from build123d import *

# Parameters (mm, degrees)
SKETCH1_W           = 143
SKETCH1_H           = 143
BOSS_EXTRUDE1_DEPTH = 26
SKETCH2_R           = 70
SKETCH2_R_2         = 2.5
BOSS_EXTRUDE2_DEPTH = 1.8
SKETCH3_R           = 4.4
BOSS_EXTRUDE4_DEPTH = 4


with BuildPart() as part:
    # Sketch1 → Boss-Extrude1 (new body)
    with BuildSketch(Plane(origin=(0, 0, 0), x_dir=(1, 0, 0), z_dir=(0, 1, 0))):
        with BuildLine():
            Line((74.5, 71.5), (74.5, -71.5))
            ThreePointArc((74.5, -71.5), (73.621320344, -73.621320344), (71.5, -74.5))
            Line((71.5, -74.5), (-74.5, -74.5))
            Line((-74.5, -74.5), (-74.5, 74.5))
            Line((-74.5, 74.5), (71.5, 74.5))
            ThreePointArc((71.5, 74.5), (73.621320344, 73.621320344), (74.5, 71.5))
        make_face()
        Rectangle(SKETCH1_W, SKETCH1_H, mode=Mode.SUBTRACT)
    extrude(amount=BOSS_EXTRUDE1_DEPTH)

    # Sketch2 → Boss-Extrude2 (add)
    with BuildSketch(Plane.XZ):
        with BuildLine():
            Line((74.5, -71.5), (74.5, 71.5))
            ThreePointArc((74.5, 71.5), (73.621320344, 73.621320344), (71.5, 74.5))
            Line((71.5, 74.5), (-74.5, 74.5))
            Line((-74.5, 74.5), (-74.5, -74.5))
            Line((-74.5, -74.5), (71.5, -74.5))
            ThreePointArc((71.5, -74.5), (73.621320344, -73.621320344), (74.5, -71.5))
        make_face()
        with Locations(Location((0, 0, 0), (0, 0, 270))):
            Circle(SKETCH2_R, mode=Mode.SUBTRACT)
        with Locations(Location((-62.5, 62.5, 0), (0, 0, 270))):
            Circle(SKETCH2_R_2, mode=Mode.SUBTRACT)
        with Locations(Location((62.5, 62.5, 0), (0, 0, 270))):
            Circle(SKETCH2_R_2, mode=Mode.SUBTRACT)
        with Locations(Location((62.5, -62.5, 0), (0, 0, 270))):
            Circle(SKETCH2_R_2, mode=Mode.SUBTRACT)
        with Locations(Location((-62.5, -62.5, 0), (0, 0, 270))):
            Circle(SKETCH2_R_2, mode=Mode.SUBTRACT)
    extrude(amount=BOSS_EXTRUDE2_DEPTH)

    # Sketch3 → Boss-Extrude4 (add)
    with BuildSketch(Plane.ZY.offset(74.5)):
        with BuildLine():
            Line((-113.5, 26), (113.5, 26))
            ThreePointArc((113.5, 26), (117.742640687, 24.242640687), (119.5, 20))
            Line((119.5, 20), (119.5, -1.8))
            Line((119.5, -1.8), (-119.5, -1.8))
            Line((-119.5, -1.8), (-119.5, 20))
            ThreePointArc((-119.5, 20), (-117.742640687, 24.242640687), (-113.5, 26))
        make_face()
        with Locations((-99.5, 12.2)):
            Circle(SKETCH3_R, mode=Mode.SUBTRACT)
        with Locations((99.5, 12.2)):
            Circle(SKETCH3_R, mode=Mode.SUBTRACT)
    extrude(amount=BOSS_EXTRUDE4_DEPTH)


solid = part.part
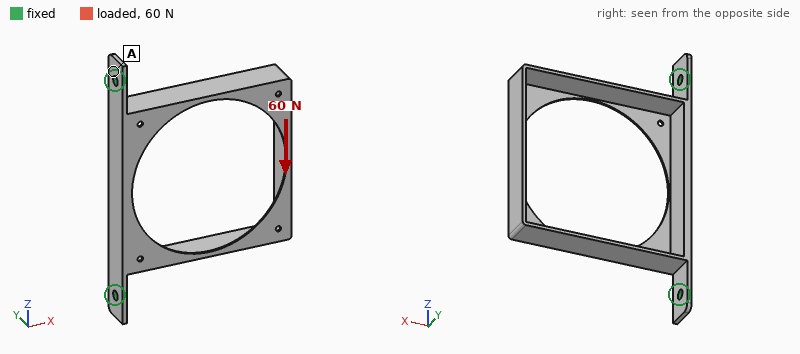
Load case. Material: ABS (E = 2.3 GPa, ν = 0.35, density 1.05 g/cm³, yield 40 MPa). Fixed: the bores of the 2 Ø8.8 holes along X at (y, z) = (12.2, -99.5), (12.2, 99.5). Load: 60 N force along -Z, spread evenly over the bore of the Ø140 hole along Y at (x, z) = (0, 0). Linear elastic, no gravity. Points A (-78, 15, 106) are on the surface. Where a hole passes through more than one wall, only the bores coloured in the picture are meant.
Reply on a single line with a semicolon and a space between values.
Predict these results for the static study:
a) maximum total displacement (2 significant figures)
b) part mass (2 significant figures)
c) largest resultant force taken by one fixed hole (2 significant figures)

2.8 mm; 88 g; 40 N
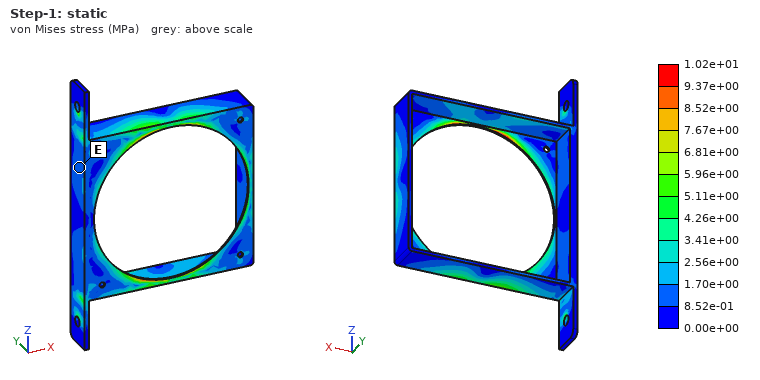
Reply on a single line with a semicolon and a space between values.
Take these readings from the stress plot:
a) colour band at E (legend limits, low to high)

8.52e-01 to 1.70e+00 MPa
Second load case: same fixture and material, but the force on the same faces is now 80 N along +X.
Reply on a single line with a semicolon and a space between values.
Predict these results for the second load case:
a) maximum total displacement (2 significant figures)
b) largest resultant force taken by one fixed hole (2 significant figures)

3.1 mm; 63 N
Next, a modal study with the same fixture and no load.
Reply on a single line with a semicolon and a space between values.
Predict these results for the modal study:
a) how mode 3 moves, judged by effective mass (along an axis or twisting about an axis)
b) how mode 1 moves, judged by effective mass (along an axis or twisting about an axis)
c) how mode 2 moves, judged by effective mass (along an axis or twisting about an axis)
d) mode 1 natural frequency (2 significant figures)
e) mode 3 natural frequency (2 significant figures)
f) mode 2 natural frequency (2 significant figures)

along Z; along Y; along Z; 48 Hz; 140 Hz; 84 Hz
